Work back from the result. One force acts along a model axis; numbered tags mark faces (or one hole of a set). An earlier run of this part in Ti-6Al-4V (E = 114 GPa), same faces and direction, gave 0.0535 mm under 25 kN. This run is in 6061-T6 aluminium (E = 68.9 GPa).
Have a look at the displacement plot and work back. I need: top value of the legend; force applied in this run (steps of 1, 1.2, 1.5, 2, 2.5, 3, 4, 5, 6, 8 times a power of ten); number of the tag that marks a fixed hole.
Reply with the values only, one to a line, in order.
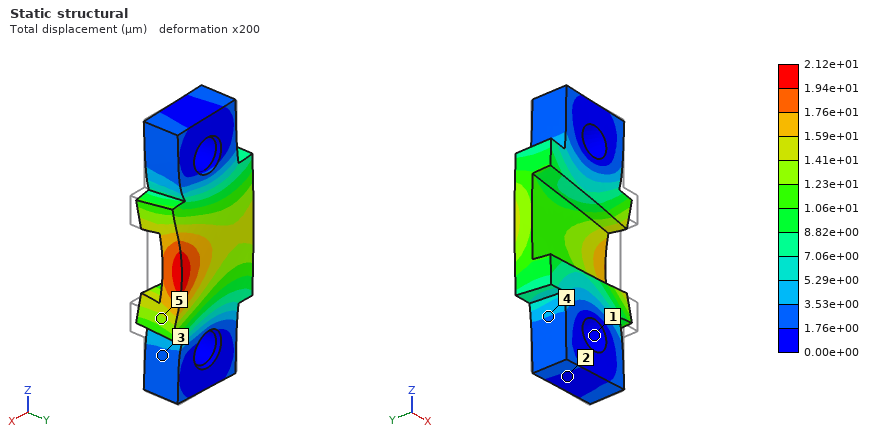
2.12e+01 µm
6 kN
1
